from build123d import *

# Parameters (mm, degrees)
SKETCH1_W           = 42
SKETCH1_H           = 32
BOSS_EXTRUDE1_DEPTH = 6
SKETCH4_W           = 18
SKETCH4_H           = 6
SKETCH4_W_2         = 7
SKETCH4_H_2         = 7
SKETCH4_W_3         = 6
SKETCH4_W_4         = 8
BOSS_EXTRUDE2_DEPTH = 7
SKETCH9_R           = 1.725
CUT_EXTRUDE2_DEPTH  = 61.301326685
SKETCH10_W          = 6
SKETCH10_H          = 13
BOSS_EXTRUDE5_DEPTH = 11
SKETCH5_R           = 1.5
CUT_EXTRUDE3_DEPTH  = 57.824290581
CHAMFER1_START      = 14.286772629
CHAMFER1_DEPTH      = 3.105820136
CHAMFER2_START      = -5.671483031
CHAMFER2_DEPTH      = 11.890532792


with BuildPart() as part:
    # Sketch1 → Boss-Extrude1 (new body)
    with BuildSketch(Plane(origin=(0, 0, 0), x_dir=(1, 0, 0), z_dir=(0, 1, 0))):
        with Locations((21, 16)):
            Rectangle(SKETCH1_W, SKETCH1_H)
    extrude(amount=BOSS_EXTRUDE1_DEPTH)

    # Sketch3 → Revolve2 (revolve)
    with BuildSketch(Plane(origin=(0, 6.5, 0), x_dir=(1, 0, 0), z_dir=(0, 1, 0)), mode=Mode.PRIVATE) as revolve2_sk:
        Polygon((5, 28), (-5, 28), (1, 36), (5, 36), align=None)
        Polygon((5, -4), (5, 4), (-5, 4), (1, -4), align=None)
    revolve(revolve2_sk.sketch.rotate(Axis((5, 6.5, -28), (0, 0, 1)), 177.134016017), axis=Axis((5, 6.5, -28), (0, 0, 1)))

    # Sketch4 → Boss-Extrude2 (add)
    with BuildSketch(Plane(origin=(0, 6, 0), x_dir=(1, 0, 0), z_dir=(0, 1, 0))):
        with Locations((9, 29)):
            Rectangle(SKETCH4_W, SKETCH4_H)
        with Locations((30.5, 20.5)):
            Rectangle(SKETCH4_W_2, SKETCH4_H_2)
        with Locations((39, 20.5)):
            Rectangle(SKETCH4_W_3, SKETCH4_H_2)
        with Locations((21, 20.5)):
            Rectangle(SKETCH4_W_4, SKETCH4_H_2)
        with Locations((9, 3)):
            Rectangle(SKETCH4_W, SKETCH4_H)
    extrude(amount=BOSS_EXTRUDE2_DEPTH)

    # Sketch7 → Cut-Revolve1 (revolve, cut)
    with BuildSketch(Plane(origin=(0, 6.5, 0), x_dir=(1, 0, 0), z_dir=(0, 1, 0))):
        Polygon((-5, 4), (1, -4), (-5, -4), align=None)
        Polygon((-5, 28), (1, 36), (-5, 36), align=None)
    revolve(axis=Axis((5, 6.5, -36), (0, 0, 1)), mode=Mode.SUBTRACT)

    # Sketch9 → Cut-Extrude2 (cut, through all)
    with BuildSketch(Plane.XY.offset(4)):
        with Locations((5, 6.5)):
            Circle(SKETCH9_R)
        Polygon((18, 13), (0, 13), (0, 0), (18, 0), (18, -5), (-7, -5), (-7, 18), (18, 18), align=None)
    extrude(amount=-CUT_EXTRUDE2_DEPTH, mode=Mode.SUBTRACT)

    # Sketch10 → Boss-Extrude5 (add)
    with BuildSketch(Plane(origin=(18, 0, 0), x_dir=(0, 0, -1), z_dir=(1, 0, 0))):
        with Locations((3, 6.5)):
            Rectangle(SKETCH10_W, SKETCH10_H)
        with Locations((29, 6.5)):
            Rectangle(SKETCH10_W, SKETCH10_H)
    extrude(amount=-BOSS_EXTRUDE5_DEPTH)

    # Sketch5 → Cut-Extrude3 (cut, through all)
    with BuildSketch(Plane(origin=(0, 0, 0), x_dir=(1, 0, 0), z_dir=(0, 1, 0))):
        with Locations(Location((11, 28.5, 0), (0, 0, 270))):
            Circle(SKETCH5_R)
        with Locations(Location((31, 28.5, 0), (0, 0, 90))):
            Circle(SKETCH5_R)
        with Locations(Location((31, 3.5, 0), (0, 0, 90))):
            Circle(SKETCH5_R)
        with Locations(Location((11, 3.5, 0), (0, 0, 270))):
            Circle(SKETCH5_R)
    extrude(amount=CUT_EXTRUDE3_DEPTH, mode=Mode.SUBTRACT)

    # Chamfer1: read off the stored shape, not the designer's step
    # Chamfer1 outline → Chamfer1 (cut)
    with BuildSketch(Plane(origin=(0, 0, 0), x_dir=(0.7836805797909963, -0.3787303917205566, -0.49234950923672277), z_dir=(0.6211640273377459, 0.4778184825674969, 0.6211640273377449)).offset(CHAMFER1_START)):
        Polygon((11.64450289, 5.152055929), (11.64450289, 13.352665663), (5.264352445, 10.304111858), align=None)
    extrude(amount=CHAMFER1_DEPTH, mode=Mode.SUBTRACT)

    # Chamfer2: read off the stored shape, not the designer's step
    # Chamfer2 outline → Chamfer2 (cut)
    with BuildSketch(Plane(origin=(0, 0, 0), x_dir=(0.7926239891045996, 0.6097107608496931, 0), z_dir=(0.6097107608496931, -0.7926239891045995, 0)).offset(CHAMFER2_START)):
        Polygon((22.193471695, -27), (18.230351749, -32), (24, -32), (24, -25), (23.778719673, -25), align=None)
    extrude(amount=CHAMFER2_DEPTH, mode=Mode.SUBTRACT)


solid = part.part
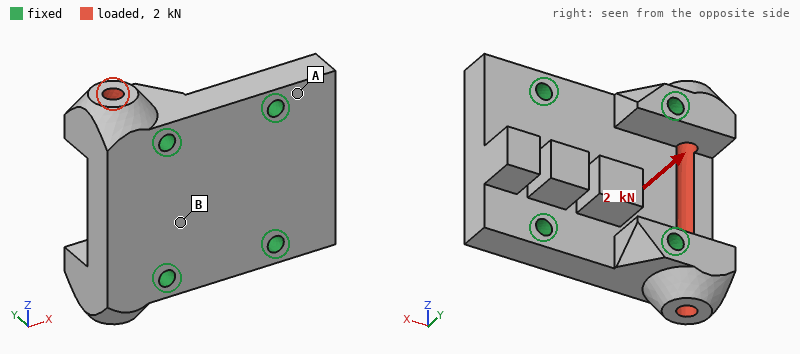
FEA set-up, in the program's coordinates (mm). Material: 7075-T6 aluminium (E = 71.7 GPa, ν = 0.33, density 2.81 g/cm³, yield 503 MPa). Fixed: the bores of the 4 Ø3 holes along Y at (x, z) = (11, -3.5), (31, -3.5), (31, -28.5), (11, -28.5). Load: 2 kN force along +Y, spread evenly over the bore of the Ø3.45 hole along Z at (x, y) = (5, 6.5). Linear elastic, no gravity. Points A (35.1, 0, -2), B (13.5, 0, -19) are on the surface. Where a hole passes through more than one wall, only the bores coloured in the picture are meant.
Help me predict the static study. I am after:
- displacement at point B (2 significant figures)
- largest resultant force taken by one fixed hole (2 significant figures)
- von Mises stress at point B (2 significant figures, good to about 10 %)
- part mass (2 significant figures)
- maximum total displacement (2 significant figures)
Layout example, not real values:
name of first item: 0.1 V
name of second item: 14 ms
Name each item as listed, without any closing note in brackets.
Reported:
displacement at point B: 1.4 µm
largest resultant force taken by one fixed hole: 1.0 kN
von Mises stress at point B: 8.4 MPa
part mass: 30 g
maximum total displacement: 7.1 µm
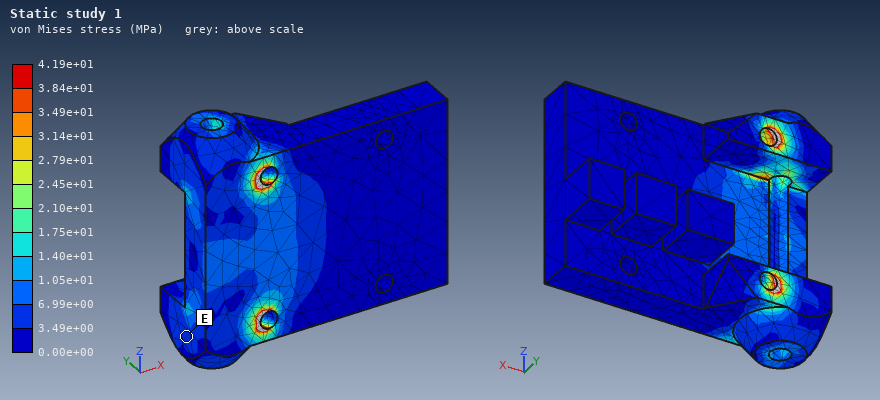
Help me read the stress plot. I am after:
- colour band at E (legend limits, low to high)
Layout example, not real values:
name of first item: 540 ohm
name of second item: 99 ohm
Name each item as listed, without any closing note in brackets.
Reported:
colour band at E: 3.49e+00 to 6.99e+00 MPa
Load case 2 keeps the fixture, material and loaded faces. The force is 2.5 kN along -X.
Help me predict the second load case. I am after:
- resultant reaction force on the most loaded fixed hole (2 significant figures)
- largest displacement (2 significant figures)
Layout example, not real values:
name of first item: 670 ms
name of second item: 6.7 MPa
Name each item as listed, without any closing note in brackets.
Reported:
resultant reaction force on the most loaded fixed hole: 1.1 kN
largest displacement: 3.9 µm
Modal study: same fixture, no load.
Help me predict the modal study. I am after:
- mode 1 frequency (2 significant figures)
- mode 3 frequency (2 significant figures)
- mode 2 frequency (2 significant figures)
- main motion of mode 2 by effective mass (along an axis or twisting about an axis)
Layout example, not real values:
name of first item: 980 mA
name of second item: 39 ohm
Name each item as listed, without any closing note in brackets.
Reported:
mode 1 frequency: 21 kHz
mode 3 frequency: 32 kHz
mode 2 frequency: 30 kHz
main motion of mode 2 by effective mass: along Y
